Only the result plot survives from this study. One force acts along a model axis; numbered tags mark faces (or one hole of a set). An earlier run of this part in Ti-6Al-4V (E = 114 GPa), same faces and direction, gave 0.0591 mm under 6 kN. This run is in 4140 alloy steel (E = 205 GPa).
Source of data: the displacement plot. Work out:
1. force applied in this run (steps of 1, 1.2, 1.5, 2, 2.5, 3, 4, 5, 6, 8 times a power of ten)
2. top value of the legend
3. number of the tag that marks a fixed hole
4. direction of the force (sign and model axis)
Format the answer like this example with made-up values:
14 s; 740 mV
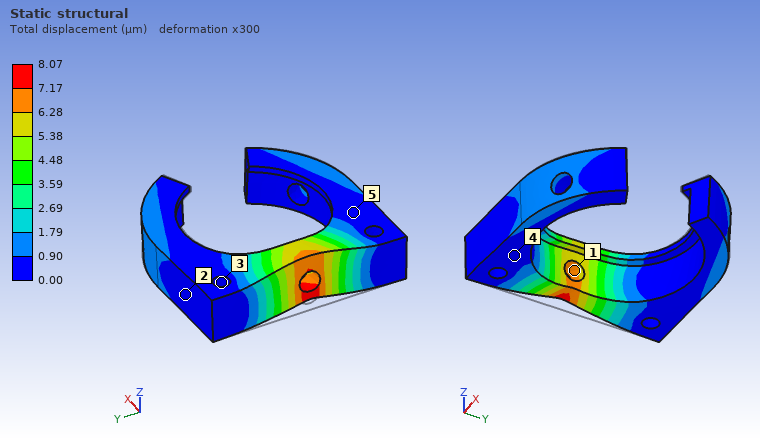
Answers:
1.5 kN; 8.07 µm; 3; +Z
